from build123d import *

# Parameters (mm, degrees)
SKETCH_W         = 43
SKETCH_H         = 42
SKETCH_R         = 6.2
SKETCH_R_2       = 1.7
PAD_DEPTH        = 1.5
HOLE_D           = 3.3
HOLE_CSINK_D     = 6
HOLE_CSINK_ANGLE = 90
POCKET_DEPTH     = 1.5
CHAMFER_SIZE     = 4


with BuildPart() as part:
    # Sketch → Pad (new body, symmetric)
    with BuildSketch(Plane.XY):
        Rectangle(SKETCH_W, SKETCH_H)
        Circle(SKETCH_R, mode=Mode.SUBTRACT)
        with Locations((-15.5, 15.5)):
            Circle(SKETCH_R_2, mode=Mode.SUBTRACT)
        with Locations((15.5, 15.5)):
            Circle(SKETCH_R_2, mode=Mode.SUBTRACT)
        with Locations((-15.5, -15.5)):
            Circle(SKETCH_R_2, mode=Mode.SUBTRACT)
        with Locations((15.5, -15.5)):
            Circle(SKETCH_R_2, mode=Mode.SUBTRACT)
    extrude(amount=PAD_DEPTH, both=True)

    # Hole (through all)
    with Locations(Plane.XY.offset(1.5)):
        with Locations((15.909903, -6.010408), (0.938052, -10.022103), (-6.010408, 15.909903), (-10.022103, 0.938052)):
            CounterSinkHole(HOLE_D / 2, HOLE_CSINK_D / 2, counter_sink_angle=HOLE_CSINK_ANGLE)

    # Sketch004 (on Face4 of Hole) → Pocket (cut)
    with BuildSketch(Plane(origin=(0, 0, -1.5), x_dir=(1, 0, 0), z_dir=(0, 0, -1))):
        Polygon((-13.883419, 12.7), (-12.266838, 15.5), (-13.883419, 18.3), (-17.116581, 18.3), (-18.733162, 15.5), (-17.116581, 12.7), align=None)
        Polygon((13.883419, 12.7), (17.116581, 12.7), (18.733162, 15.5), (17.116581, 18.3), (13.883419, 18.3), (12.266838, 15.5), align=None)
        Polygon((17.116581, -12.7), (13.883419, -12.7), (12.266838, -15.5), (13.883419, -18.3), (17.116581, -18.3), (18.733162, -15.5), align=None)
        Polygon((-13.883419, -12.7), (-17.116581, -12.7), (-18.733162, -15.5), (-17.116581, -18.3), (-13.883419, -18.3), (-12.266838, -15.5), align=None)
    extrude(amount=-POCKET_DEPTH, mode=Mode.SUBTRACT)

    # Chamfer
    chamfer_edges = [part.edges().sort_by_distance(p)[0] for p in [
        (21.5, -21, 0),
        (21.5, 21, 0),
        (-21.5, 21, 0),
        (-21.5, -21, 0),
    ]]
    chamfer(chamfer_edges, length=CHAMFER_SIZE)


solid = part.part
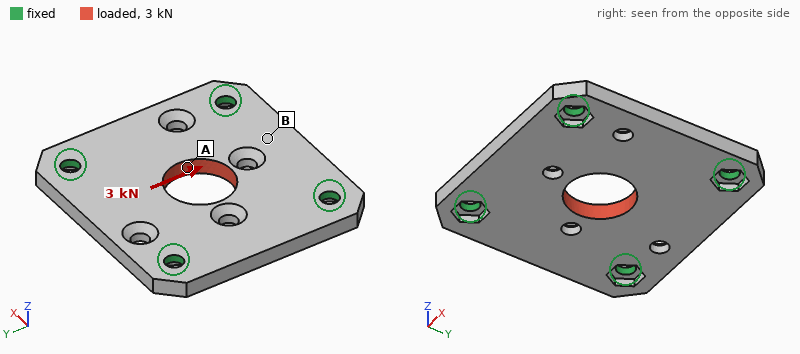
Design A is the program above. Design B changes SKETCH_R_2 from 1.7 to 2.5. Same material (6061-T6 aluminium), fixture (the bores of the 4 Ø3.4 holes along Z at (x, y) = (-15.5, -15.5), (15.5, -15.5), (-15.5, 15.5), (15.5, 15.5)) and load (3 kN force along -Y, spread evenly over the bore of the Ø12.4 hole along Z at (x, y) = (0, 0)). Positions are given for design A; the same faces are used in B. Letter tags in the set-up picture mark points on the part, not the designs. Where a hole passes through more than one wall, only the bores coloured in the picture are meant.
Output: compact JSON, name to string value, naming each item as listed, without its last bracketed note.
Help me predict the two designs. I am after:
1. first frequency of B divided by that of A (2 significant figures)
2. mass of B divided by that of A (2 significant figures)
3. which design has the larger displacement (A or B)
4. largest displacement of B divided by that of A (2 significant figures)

{"first frequency of B divided by that of A": "1.2", "mass of B divided by that of A": "0.99", "which design has the larger displacement": "A", "largest displacement of B divided by that of A": "0.87"}
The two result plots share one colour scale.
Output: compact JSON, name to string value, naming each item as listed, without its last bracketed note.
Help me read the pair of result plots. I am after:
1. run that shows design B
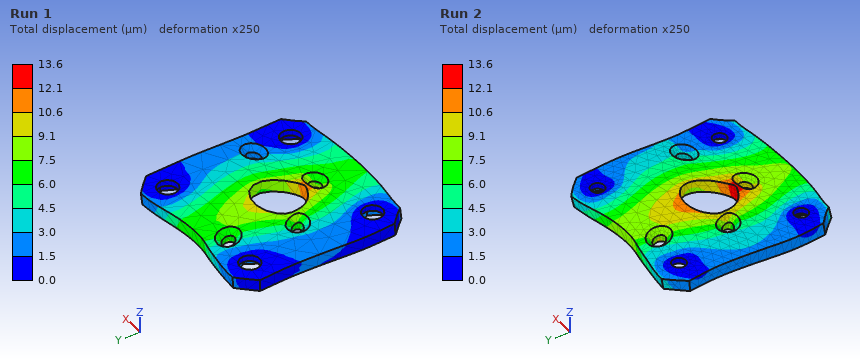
{"run that shows design B": "Run 1"}
